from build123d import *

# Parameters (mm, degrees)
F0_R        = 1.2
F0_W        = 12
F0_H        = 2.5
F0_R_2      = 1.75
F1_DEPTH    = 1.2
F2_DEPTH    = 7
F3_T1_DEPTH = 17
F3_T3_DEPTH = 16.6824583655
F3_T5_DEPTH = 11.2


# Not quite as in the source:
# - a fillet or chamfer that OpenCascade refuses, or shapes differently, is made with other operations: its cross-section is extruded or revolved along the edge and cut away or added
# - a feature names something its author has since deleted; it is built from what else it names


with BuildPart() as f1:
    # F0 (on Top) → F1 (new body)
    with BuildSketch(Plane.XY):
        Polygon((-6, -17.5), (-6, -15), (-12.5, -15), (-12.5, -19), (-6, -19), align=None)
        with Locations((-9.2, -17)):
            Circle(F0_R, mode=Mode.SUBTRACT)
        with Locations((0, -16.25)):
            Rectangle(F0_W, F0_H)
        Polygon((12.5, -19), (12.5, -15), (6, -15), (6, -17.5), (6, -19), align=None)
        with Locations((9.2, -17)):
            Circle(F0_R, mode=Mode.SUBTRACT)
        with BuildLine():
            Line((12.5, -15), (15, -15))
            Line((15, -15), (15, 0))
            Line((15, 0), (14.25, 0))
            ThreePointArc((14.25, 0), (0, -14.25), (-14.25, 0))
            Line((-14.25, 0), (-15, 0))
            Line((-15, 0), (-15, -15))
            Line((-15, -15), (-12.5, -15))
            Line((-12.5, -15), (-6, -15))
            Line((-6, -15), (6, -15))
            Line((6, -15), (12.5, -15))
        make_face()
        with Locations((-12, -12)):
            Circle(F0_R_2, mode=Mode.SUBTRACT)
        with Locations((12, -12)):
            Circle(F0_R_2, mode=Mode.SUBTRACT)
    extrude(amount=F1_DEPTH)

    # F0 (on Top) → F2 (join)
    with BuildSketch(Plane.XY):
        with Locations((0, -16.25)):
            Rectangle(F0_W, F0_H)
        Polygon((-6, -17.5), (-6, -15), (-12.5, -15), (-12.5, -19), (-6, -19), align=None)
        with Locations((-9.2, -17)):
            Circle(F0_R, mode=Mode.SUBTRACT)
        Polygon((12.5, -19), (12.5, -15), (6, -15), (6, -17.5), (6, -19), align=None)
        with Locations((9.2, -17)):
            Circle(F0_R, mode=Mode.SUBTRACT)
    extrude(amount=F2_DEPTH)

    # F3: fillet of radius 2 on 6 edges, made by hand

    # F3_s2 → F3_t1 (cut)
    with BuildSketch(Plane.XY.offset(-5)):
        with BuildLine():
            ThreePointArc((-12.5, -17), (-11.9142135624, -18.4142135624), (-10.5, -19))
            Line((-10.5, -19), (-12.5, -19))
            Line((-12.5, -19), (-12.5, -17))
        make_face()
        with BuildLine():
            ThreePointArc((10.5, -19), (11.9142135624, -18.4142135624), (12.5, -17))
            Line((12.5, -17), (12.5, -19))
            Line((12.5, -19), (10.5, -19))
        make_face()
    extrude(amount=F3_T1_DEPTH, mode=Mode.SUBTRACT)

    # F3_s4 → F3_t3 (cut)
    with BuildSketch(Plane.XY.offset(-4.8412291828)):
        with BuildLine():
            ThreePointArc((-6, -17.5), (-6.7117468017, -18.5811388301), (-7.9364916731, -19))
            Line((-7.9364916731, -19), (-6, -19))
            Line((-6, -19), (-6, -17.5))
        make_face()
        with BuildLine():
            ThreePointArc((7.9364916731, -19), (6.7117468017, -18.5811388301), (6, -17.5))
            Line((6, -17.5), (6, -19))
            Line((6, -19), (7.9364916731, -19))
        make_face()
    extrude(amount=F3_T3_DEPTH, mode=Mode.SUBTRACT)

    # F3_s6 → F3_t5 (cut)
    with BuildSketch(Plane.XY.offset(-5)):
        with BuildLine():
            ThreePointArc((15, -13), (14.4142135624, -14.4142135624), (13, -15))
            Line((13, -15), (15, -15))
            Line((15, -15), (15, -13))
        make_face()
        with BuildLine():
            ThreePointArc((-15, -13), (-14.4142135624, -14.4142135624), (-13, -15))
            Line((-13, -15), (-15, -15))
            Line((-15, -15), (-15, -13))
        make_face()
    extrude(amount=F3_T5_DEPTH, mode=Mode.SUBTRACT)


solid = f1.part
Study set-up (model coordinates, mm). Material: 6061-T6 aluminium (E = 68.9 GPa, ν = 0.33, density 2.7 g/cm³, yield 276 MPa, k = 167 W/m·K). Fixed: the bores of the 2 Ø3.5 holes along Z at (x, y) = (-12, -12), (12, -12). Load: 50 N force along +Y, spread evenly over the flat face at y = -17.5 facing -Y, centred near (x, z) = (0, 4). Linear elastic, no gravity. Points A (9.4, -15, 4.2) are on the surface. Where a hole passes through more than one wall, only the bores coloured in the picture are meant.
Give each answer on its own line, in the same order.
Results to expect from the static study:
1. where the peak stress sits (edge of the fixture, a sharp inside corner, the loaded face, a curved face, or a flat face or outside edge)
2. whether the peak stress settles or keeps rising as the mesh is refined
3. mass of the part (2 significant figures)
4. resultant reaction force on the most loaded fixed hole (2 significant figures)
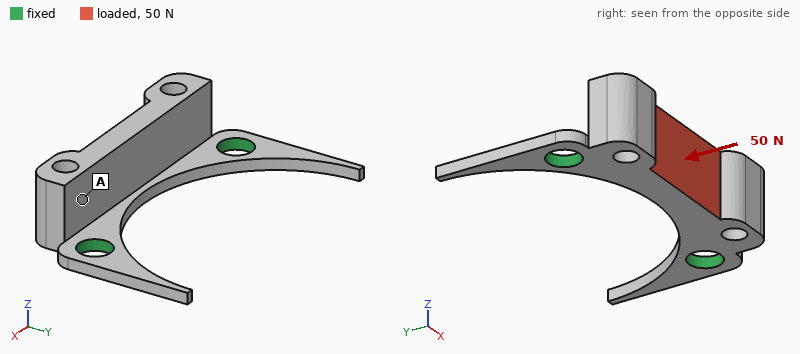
a sharp inside corner
keeps rising
1.7 g
34 N
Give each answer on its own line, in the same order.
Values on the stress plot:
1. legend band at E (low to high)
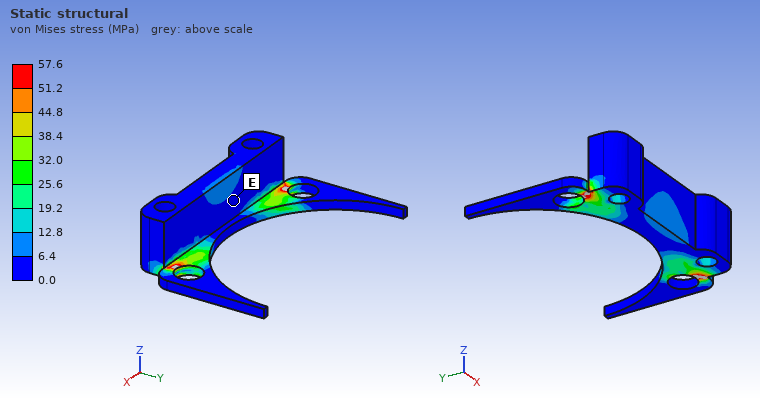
0.0 to 6.4 MPa
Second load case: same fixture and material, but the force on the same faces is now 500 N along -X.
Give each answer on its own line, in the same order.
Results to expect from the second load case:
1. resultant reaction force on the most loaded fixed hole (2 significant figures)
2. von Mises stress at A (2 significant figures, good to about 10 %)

270 N
13 MPa
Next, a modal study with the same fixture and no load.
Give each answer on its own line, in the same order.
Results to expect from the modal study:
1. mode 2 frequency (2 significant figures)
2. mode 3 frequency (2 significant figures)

15 kHz
15 kHz
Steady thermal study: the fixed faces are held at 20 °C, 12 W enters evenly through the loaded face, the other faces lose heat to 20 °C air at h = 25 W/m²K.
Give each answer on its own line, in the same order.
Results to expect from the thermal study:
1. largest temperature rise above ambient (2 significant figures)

29 K
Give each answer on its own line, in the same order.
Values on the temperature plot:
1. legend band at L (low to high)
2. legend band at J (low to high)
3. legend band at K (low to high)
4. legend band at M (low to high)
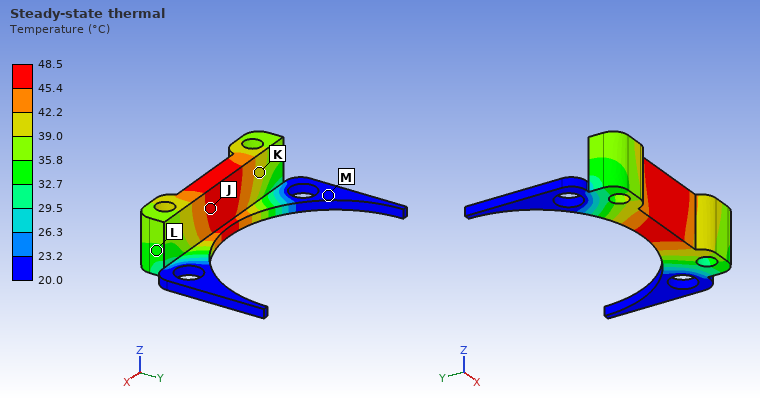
32.7 to 35.8 °C
45.4 to 48.5 °C
39.0 to 42.2 °C
20.0 to 23.2 °C
